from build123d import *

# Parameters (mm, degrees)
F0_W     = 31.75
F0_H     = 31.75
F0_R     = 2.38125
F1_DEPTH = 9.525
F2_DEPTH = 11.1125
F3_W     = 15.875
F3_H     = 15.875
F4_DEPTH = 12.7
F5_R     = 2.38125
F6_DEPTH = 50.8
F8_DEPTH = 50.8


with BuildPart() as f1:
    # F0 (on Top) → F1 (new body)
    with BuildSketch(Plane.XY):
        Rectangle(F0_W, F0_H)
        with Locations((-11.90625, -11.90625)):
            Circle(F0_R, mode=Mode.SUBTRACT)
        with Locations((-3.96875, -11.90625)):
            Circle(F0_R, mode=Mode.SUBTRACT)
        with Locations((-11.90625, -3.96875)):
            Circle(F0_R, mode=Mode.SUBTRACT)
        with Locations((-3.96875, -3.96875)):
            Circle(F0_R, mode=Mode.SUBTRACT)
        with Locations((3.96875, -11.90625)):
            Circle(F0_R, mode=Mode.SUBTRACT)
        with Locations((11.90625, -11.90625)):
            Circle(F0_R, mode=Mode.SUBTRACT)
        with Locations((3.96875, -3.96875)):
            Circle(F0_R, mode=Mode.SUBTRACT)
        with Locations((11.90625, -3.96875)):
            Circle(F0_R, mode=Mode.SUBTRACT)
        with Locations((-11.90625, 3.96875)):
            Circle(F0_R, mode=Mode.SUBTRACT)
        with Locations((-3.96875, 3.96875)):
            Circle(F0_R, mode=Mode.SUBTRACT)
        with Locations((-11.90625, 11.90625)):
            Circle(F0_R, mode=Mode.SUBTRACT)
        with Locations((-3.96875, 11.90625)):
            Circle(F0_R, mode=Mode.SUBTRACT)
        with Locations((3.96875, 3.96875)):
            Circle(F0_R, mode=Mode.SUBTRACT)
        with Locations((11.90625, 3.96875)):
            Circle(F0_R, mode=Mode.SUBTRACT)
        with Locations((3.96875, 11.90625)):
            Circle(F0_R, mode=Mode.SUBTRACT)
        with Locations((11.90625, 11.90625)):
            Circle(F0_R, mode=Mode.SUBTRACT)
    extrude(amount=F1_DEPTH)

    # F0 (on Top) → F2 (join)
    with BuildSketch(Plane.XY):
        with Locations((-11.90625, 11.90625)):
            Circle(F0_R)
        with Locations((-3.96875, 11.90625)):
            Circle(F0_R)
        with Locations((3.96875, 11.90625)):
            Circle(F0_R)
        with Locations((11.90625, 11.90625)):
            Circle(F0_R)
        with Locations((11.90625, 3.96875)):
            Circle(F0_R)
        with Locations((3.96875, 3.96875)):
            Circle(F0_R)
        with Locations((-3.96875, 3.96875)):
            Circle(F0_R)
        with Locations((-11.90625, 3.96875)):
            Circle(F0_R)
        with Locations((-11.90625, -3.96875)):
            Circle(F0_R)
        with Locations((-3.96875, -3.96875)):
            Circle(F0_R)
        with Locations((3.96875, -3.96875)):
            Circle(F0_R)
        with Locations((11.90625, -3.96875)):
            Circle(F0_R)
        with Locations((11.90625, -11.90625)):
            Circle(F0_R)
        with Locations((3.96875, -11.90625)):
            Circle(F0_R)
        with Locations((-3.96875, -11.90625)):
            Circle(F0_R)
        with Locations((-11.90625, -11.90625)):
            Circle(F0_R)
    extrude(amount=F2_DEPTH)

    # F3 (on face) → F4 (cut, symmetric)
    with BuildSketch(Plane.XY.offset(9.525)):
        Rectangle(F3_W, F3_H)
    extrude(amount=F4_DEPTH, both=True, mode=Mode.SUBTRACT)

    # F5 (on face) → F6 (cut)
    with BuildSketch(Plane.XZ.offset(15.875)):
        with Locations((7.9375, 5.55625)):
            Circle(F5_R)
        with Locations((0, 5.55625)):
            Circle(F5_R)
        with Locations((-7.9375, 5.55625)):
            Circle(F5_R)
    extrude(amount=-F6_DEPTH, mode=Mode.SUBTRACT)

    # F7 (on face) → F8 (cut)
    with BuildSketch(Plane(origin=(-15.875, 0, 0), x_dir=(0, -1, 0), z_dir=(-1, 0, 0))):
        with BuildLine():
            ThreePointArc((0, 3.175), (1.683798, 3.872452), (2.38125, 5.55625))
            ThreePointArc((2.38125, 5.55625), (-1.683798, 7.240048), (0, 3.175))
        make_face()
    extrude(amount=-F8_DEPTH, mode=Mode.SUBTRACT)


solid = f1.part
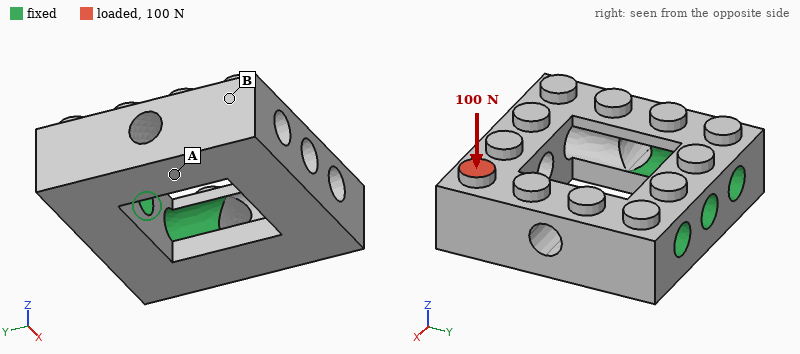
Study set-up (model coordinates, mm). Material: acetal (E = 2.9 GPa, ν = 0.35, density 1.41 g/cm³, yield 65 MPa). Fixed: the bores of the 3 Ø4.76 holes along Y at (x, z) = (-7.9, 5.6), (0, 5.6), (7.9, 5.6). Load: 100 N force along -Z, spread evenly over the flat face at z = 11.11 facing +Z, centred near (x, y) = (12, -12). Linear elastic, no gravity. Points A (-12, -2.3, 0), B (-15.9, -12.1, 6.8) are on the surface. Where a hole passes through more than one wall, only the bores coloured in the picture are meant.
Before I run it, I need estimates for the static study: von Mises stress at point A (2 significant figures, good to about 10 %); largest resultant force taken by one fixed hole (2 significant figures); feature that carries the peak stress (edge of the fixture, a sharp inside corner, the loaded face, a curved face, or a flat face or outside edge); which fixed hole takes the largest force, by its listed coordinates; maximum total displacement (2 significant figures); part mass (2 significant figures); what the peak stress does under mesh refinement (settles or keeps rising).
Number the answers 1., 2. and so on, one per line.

1. 4.1 MPa
2. 91 N
3. edge of the fixture
4. (7.9, 5.6)
5. 0.19 mm
6. 8.7 g
7. keeps rising
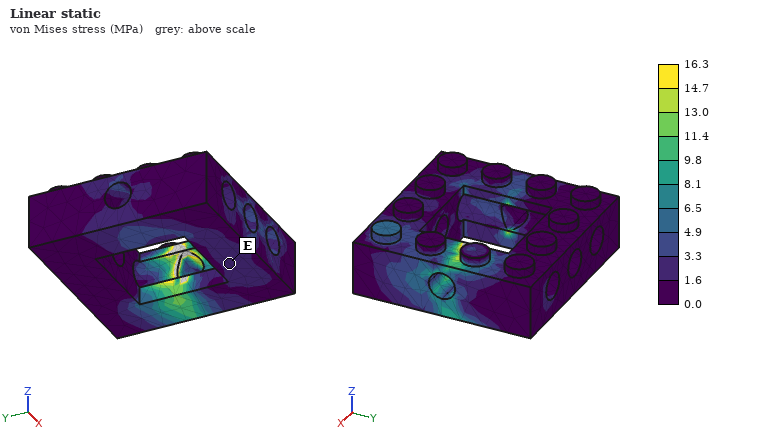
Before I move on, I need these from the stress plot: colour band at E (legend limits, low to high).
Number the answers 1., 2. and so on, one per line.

1. 1.6 to 3.3 MPa
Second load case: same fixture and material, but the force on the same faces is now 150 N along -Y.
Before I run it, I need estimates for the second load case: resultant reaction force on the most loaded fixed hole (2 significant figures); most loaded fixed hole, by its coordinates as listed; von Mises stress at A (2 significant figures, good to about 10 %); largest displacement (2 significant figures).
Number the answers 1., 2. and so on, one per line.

1. 150 N
2. (7.9, 5.6)
3. 2.7 MPa
4. 0.16 mm
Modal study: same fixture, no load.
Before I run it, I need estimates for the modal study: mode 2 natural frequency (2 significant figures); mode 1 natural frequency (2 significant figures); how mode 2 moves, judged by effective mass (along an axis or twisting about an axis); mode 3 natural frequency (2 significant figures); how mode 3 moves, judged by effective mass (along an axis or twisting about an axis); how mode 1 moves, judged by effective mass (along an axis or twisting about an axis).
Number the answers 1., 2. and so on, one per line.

1. 3900 Hz
2. 2800 Hz
3. along X
4. 4200 Hz
5. twisting about Y
6. along Z
